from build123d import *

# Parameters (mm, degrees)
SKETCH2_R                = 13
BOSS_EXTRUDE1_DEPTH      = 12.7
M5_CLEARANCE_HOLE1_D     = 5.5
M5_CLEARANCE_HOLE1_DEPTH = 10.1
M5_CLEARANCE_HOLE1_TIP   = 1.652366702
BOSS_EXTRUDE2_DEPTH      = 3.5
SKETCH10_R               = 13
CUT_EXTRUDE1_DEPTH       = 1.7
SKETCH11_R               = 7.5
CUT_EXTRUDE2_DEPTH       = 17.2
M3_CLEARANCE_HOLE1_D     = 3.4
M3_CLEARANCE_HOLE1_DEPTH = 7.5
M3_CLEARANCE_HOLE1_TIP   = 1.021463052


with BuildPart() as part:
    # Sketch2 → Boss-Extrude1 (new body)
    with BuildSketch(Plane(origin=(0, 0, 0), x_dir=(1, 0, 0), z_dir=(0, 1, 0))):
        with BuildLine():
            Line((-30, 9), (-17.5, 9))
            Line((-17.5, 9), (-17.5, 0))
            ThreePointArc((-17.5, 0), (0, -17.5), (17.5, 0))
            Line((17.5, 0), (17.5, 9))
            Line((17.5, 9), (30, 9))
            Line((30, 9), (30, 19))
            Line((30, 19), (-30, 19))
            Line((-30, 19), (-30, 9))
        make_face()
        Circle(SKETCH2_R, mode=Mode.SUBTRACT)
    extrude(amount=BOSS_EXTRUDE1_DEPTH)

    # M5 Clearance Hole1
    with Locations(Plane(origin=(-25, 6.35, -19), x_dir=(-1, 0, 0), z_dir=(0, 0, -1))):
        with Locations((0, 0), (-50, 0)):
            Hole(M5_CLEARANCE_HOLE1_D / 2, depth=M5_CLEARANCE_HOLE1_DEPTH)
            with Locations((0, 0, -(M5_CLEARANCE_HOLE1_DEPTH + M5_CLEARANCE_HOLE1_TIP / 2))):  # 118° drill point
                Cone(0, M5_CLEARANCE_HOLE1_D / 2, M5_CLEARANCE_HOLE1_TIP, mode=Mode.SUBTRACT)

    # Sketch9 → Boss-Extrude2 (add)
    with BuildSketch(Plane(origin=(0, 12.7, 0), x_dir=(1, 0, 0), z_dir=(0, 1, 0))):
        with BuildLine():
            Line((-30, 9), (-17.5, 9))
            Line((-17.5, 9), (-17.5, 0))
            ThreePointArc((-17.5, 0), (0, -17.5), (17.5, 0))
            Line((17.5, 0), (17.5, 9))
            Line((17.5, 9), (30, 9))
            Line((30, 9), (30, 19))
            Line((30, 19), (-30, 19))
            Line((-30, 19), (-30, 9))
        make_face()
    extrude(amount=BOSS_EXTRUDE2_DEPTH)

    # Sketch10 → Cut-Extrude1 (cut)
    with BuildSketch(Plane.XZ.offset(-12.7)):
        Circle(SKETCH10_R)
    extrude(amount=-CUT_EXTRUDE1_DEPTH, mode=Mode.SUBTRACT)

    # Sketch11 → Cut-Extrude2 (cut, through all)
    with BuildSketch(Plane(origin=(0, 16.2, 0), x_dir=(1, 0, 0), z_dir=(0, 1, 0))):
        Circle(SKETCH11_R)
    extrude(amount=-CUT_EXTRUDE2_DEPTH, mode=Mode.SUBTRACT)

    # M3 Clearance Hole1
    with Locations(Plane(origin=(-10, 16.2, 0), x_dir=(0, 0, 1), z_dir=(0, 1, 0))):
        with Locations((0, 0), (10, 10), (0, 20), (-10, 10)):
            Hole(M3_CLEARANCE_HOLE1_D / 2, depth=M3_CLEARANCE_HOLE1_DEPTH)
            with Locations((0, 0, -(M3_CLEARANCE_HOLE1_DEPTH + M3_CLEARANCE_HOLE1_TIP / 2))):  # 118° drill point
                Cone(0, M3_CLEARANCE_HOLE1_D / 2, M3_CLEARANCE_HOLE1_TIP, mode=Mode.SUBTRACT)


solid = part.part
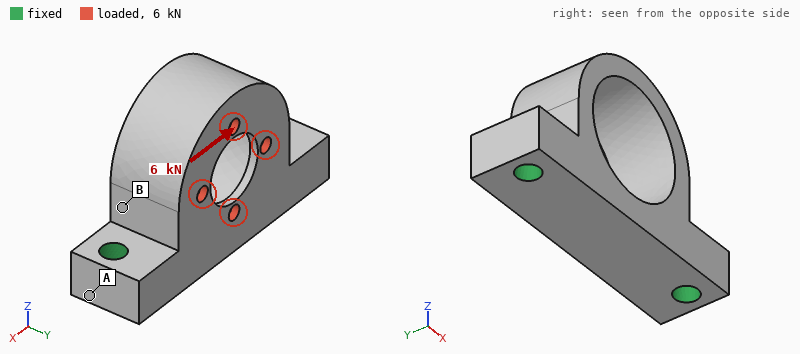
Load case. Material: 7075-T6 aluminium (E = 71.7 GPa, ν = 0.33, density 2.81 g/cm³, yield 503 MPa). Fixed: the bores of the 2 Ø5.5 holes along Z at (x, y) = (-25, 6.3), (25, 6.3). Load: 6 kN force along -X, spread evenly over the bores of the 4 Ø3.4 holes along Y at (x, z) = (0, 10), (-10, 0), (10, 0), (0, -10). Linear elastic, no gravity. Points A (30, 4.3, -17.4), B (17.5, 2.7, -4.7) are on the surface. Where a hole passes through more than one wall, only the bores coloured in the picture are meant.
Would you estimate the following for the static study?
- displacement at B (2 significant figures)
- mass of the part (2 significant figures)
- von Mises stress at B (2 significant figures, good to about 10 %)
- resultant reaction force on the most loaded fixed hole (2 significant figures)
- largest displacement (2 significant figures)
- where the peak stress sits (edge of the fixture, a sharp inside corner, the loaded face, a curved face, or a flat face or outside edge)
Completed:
17 µm
40 g
85 MPa
3.7 kN
85 µm
the loaded face
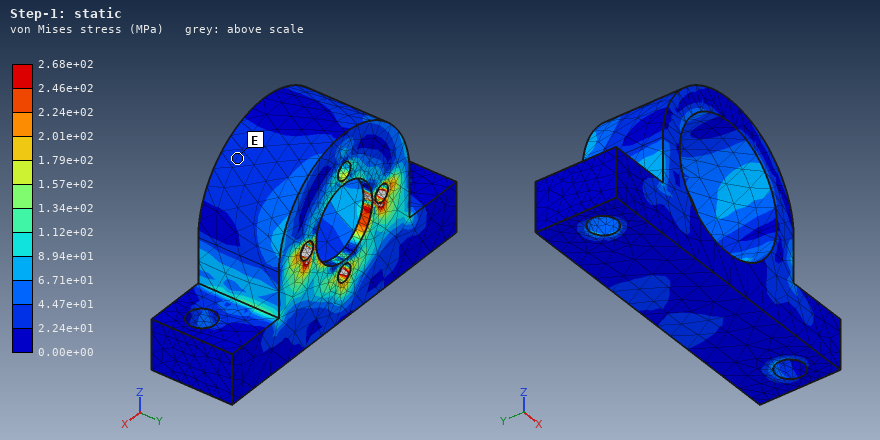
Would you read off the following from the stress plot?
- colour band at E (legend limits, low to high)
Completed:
2.24e+01 to 4.47e+01 MPa
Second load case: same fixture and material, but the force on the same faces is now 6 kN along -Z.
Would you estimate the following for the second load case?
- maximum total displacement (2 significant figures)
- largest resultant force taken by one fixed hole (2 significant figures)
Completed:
0.13 mm
3.0 kN
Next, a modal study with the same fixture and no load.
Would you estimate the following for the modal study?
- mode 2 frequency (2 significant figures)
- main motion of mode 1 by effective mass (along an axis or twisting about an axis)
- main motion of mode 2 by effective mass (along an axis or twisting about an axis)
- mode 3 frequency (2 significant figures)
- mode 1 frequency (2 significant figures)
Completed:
9800 Hz
along Y
along X
16 kHz
6700 Hz
